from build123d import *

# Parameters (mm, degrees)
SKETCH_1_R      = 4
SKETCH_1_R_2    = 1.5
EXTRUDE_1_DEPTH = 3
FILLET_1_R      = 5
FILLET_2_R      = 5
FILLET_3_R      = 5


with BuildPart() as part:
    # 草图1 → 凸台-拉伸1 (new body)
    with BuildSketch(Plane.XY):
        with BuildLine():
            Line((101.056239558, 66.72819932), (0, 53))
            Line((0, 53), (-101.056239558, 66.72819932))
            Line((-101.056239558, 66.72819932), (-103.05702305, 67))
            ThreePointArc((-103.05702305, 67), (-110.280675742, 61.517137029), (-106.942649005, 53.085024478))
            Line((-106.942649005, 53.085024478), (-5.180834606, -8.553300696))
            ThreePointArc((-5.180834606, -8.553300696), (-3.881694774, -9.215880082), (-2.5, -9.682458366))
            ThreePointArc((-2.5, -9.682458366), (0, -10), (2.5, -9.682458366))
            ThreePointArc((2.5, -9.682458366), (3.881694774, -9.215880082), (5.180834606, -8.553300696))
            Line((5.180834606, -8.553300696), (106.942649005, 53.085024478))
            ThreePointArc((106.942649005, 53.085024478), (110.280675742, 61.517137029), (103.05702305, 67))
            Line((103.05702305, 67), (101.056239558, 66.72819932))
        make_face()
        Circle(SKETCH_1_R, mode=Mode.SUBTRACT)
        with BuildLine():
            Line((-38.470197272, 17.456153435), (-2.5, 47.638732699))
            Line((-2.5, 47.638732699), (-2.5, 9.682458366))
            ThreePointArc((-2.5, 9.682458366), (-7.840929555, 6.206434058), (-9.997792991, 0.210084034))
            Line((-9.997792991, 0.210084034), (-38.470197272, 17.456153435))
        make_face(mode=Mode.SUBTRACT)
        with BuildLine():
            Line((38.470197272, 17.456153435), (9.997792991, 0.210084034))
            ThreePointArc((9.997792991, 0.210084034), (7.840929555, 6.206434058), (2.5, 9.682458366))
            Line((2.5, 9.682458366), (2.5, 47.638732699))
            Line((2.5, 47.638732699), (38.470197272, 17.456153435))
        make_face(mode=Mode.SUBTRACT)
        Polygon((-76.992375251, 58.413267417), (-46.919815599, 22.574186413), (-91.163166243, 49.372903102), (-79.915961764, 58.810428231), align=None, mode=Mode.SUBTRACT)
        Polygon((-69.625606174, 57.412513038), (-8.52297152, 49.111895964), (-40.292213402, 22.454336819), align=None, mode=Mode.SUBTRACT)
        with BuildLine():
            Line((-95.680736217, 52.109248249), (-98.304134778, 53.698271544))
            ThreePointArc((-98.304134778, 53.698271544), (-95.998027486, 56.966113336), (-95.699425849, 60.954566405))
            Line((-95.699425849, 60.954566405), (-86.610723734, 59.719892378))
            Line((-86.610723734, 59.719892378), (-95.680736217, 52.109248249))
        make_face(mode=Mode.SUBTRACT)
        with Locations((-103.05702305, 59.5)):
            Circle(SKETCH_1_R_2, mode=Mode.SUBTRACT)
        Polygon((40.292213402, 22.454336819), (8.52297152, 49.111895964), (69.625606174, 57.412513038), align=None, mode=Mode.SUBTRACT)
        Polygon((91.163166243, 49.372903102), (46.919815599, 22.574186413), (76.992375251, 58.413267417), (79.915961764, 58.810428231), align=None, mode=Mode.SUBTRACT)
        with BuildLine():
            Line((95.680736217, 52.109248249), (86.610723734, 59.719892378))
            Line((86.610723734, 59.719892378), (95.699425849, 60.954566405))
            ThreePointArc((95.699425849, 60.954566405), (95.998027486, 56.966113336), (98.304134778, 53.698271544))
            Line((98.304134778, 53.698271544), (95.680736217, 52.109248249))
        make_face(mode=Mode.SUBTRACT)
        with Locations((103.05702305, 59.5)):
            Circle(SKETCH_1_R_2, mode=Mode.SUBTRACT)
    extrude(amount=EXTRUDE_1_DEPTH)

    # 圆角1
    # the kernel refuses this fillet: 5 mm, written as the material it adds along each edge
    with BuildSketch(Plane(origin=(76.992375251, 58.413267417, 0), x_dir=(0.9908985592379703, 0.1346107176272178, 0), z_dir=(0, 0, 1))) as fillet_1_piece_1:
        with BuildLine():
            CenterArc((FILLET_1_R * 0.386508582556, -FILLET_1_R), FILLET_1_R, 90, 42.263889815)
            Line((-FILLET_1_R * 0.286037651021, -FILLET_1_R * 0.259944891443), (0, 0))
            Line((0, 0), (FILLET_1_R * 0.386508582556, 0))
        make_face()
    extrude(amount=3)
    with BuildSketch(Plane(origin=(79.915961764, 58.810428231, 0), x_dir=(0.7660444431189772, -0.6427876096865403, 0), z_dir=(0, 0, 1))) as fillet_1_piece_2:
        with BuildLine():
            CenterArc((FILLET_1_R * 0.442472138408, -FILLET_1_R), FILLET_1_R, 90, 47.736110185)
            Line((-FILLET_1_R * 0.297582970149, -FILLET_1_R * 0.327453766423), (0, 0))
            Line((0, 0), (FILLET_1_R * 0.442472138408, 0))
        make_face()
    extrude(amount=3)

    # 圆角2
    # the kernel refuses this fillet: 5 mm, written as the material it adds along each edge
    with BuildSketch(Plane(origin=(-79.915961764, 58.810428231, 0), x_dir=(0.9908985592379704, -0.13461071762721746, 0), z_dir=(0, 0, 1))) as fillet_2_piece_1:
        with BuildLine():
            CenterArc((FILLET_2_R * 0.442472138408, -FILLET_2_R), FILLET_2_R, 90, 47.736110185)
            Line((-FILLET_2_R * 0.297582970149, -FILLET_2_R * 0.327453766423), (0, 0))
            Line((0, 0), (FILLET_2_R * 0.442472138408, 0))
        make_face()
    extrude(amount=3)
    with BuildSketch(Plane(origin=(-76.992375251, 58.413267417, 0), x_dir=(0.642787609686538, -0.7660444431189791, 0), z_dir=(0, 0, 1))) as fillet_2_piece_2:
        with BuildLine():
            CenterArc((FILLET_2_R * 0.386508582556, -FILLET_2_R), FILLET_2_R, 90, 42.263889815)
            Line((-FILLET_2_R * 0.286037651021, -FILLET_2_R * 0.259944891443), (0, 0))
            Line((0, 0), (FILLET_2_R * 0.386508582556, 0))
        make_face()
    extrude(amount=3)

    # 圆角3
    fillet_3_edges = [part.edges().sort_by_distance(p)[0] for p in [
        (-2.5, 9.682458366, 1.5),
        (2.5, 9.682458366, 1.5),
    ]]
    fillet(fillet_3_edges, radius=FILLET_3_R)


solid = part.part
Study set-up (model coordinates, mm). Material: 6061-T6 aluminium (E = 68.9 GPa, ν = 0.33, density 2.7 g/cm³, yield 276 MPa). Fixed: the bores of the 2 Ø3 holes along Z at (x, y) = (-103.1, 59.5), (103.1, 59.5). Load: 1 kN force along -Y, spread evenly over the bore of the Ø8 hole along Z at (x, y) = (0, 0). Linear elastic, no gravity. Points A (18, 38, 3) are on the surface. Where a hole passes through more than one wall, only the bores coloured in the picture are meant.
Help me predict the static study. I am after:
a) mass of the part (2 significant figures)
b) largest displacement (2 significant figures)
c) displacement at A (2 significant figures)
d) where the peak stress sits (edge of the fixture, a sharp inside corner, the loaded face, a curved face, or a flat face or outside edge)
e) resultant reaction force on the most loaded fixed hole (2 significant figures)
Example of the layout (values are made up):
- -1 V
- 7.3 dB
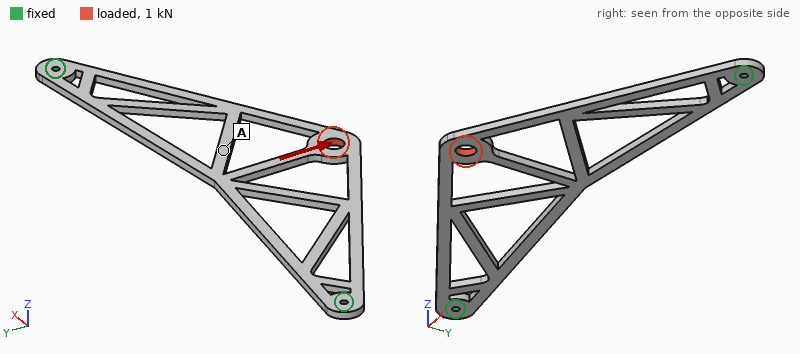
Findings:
- 32 g
- 0.15 mm
- 0.13 mm
- edge of the fixture
- 870 N
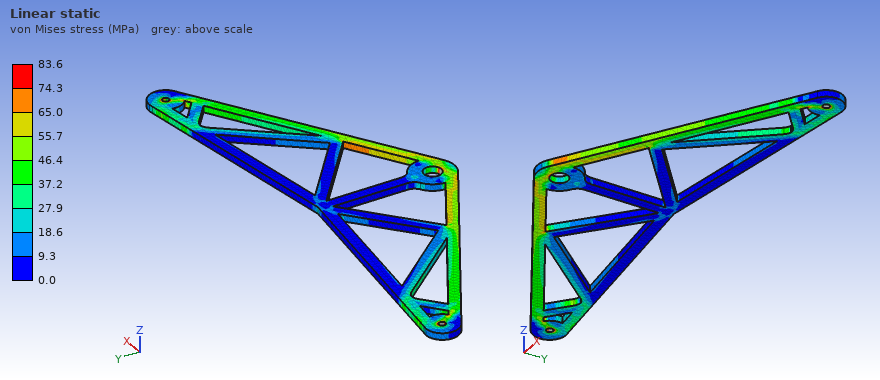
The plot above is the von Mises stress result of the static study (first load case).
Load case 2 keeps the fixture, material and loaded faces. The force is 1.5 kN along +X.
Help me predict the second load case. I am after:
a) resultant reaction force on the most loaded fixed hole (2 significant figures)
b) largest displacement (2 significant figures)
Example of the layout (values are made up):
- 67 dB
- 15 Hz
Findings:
- 870 N
- 0.26 mm
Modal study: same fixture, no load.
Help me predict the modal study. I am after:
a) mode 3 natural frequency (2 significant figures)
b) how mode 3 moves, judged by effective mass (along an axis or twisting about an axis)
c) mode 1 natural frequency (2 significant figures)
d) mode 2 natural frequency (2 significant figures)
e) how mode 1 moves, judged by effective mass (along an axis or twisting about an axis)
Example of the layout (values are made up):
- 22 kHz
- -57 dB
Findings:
- 730 Hz
- twisting about Y
- 220 Hz
- 550 Hz
- along Z
